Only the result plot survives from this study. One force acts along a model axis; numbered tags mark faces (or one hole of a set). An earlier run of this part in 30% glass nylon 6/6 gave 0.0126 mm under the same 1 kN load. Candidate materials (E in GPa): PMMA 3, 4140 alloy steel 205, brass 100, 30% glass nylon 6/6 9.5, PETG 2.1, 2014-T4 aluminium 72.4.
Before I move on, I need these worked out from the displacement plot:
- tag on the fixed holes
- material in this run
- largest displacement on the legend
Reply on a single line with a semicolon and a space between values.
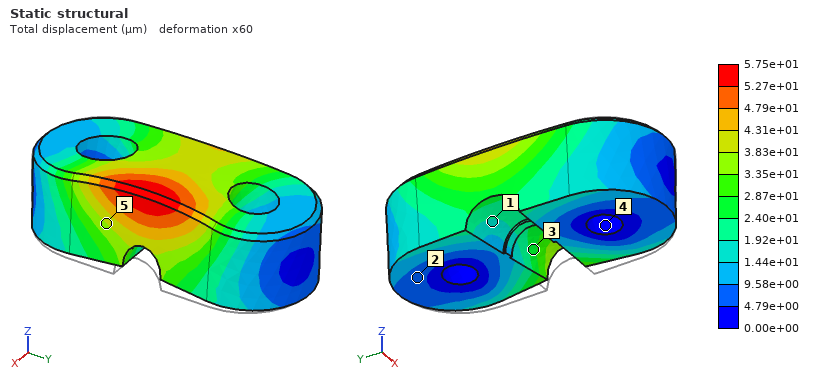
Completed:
4; PETG; 5.75e+01 µm
